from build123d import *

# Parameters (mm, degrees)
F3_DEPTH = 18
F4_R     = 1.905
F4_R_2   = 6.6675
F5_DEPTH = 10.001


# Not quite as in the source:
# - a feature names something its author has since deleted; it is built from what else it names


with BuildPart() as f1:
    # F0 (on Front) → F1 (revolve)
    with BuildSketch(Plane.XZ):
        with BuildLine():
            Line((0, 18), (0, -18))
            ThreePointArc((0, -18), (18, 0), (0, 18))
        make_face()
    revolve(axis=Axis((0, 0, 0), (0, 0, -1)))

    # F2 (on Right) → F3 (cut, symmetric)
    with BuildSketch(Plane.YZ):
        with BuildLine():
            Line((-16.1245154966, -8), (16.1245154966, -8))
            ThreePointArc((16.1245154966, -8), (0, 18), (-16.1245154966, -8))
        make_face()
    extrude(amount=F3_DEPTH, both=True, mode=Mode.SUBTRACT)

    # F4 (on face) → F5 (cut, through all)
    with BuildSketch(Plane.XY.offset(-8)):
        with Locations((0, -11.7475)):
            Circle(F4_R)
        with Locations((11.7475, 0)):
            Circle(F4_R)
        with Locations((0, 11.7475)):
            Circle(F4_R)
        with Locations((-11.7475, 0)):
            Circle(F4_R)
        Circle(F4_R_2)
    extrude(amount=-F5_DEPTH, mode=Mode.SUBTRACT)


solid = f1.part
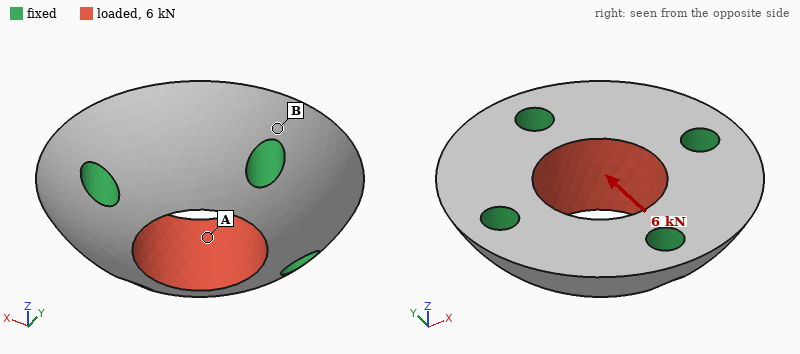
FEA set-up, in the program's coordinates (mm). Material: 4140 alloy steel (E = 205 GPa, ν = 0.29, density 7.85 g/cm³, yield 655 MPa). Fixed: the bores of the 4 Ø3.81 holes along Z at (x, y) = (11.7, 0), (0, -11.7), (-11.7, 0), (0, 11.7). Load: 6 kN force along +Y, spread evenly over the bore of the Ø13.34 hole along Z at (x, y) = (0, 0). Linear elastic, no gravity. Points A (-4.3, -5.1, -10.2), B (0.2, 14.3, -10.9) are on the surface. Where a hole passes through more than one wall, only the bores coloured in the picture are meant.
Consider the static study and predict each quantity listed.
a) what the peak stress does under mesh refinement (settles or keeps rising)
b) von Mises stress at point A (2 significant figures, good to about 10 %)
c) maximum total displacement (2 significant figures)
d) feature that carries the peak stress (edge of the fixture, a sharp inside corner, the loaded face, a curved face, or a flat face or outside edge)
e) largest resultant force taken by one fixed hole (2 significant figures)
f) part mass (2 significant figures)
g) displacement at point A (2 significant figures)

keeps rising
24 MPa
2.2 µm
edge of the fixture
1.6 kN
24 g
1.0 µm
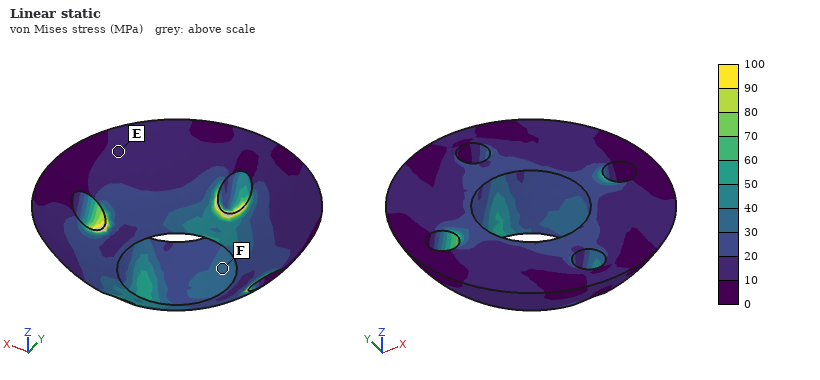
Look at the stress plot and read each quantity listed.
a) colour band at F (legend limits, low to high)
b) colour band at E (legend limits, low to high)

30 to 40 MPa
10 to 20 MPa
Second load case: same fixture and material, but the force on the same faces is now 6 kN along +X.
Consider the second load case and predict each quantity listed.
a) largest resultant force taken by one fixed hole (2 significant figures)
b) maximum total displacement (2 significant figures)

1.6 kN
2.2 µm
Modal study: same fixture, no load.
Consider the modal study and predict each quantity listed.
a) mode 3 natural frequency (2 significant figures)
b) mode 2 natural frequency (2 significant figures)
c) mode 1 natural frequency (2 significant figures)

69 kHz
69 kHz
65 kHz
